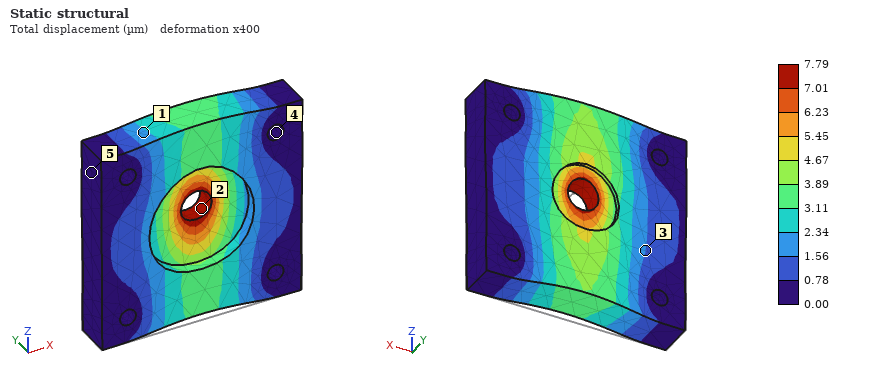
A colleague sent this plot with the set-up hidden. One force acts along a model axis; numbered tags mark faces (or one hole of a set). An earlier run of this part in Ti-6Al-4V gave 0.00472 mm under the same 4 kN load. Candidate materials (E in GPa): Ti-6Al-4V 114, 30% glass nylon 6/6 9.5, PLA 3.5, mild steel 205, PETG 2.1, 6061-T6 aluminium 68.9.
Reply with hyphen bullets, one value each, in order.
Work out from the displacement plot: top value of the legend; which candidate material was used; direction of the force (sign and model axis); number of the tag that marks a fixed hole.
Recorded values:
- 7.79 µm
- 6061-T6 aluminium
- +Z
- 4
